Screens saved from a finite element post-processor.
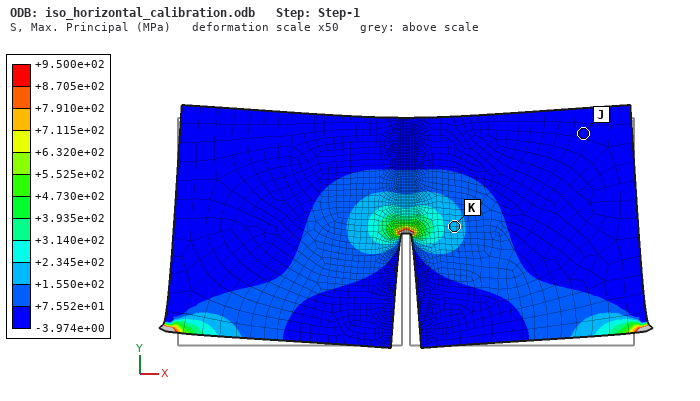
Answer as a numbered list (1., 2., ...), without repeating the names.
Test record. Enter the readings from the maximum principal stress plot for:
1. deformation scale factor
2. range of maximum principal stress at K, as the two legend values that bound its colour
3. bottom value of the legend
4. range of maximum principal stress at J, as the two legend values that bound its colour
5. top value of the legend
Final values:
1. 50
2. +1.550e+02 to +2.345e+02 MPa
3. -3.974e+00 MPa
4. -3.974e+00 to +7.552e+01 MPa
5. +9.500e+02 MPa
